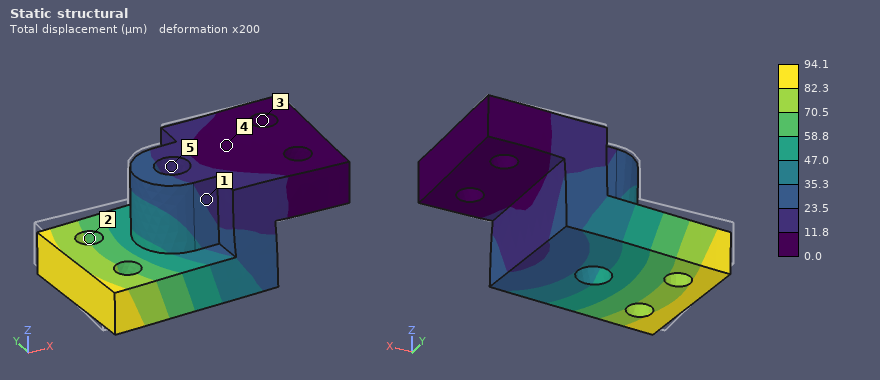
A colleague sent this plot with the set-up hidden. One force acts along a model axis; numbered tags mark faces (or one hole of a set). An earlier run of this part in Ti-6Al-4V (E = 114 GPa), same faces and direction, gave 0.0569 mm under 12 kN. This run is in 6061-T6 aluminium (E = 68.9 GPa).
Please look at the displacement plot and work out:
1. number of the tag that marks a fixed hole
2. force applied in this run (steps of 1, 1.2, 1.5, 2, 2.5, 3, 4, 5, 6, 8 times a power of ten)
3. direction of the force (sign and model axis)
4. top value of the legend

3
12 kN
-Y
94.1 µm
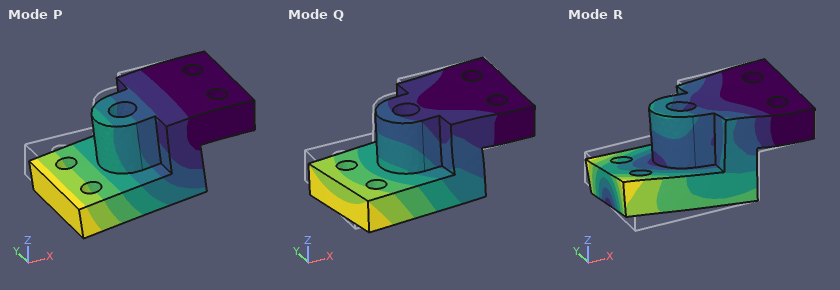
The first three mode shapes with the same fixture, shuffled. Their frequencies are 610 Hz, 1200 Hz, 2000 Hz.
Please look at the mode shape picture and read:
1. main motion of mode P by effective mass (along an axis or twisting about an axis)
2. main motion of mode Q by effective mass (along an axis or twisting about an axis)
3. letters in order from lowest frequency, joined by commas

along Z
along Y
P, Q, R
